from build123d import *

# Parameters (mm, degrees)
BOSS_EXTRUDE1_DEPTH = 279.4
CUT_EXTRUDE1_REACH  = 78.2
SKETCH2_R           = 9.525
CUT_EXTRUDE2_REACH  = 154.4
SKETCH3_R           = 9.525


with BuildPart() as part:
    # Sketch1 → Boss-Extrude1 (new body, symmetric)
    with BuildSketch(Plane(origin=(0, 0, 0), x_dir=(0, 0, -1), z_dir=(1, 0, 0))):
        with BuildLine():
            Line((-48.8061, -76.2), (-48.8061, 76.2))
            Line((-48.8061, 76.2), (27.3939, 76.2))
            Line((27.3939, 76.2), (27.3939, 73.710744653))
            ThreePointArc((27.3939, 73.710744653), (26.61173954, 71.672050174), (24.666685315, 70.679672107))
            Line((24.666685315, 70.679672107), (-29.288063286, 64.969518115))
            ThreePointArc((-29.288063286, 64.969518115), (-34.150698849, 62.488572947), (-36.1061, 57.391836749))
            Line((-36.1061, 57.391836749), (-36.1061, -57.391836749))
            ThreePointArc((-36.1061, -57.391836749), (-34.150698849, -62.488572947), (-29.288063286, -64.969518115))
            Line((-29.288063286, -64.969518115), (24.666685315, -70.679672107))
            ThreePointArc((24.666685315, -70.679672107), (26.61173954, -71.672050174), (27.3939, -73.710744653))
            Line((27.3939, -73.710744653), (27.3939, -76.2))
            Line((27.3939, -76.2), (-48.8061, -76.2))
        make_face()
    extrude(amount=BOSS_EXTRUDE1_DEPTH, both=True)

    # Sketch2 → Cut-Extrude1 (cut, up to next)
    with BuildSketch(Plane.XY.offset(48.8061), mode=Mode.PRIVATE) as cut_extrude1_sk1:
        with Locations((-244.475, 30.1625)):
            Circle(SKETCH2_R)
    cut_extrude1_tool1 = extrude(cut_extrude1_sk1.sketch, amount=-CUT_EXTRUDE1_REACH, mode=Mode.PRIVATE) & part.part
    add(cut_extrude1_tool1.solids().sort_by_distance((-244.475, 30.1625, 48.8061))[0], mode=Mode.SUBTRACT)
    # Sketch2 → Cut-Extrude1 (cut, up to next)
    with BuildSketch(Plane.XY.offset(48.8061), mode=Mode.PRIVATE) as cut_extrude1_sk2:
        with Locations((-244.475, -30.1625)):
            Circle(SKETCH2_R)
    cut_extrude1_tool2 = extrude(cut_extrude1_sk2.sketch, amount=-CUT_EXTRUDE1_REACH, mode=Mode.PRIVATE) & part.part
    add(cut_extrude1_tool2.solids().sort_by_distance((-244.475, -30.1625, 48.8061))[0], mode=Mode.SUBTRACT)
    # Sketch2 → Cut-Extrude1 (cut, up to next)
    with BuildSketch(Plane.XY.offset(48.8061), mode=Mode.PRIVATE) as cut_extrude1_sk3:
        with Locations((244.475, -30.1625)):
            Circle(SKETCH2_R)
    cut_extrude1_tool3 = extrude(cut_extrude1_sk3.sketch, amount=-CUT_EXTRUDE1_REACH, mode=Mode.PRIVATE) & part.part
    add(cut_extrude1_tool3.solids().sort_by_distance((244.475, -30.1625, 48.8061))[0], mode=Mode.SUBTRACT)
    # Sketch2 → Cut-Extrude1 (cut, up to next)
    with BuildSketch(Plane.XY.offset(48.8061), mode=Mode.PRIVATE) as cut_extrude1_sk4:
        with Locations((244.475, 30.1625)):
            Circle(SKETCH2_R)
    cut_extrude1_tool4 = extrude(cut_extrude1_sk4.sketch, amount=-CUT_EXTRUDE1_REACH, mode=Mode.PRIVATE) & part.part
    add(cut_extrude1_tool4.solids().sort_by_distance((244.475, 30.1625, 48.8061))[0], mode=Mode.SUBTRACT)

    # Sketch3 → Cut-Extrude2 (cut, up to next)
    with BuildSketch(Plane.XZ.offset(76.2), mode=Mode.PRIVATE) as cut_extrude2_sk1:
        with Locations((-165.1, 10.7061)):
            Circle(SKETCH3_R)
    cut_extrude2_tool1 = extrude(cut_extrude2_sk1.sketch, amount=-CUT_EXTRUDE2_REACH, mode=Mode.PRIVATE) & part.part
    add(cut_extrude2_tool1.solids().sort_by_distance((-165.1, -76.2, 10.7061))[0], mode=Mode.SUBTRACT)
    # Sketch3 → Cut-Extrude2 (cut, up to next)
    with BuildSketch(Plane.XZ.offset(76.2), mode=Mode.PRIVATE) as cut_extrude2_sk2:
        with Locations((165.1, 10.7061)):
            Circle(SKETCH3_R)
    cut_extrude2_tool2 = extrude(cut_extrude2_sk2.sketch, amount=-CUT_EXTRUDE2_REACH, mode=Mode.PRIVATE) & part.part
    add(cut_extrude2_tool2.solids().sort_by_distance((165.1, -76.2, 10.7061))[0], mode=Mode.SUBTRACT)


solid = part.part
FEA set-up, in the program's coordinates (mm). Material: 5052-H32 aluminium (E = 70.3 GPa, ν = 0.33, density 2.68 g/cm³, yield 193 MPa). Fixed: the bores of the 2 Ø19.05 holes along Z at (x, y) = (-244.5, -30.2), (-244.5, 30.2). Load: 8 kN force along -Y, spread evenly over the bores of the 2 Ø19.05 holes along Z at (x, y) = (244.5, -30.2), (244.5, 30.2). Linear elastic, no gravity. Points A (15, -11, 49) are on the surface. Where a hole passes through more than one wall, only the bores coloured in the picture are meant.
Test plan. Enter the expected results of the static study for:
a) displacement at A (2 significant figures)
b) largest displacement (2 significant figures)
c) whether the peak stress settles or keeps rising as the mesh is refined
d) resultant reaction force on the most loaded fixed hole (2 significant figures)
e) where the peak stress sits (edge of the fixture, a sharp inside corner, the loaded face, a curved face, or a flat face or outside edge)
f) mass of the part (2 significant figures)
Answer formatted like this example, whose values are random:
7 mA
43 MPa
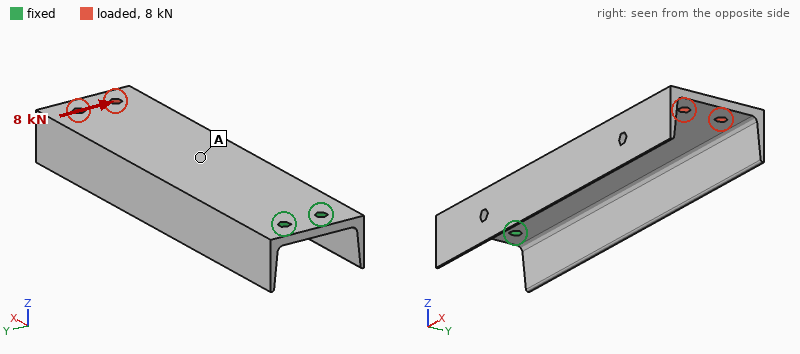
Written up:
0.54 mm
1.5 mm
keeps rising
51 kN
edge of the fixture
4.5 kg
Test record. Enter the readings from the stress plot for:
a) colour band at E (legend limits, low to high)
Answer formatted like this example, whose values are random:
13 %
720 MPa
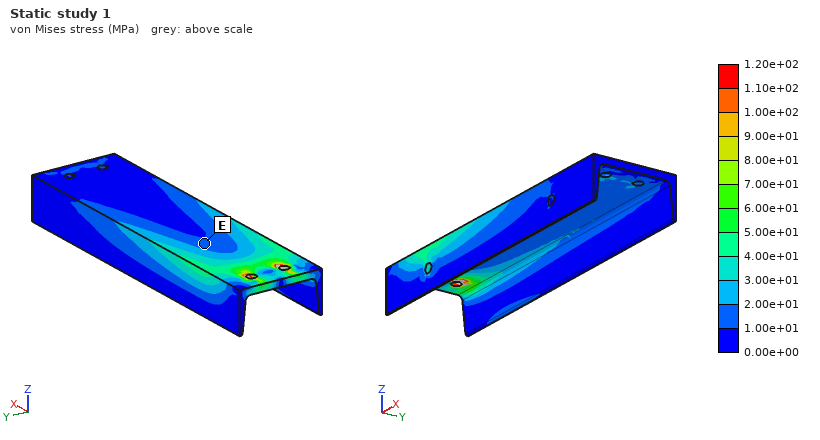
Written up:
1.00e+01 to 2.00e+01 MPa
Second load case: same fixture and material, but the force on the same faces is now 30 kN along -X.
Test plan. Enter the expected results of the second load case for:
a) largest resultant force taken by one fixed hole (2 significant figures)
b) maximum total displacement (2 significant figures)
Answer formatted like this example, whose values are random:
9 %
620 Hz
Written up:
15 kN
0.51 mm
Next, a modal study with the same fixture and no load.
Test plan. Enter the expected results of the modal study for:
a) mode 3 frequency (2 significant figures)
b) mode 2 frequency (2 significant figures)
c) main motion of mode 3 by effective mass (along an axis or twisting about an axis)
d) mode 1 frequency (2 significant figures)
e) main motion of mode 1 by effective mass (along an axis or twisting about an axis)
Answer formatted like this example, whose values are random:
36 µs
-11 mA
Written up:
340 Hz
190 Hz
along Y
86 Hz
along Z
